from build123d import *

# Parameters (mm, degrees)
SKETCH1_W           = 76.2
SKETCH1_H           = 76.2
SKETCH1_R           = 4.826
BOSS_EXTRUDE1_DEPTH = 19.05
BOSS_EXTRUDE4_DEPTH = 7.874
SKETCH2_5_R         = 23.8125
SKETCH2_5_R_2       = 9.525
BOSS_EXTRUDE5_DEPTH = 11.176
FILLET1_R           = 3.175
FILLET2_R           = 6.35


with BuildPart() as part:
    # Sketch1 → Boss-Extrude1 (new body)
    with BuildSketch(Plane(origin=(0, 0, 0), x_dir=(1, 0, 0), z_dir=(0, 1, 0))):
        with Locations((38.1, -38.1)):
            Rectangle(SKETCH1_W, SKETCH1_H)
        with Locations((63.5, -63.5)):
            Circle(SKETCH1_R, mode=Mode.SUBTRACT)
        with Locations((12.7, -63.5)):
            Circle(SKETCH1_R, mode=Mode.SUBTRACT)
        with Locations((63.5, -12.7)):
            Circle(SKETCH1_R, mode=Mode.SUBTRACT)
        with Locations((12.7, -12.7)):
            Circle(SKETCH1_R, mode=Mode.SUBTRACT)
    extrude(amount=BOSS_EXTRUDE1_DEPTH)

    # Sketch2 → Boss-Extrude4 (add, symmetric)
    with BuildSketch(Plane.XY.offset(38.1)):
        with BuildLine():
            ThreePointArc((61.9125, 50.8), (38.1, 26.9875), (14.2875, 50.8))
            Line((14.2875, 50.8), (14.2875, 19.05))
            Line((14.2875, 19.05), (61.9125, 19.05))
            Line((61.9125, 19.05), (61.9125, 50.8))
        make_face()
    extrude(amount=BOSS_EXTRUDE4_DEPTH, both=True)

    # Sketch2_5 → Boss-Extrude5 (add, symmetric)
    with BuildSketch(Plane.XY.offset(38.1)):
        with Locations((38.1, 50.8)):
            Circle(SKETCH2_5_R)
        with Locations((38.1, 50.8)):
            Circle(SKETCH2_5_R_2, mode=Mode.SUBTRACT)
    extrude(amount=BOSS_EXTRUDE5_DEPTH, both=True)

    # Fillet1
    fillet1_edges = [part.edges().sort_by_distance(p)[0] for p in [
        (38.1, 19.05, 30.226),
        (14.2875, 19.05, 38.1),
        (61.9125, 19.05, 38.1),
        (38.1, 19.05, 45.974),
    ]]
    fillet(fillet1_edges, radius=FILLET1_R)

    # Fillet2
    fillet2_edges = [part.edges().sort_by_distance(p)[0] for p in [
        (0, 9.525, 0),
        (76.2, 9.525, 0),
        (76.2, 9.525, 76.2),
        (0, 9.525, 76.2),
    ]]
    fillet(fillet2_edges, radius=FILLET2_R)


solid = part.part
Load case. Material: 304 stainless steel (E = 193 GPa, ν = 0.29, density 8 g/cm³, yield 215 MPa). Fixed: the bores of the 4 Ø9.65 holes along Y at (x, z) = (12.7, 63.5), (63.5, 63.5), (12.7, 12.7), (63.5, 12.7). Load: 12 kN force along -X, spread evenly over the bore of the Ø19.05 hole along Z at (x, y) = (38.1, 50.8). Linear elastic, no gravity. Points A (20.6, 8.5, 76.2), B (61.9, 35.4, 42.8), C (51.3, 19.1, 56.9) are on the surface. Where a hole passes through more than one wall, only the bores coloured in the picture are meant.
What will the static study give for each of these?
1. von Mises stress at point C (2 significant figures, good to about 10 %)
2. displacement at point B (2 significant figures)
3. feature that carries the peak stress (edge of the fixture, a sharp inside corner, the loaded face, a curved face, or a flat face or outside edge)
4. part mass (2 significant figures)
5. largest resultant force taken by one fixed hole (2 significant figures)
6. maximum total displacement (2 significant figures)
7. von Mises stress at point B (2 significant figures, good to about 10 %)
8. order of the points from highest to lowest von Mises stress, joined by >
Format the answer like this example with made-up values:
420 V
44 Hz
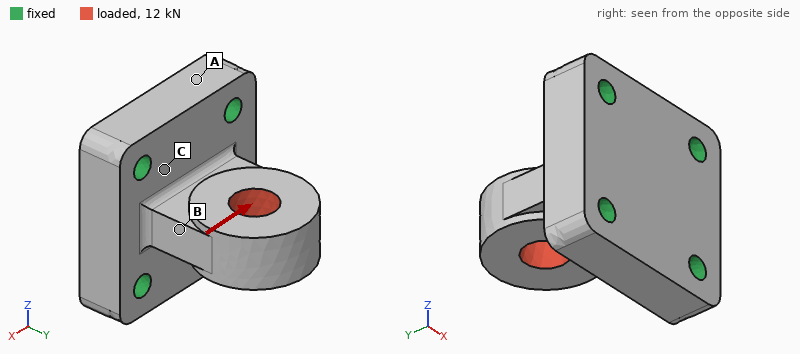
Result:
19 MPa
14 µm
a curved face
1.2 kg
5.8 kN
33 µm
39 MPa
B > C > A
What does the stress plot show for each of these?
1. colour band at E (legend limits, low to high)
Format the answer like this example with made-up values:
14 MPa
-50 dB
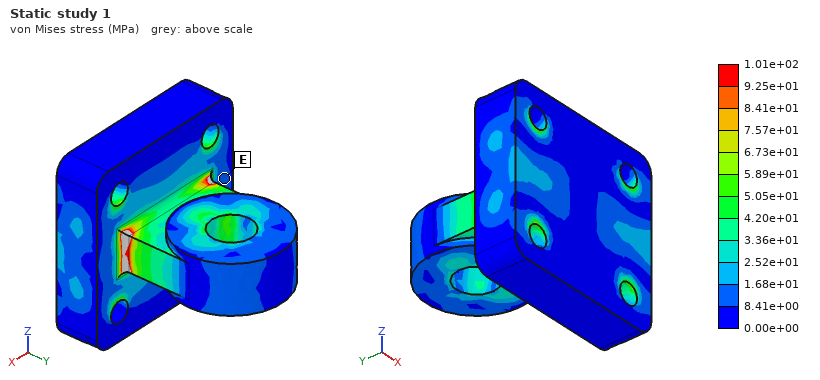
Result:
8.41e+00 to 1.68e+01 MPa
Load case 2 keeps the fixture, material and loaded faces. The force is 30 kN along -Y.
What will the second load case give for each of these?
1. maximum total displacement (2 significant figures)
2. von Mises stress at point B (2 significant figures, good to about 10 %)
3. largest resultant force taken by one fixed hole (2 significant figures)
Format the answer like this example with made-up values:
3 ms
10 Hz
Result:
17 µm
37 MPa
7.7 kN
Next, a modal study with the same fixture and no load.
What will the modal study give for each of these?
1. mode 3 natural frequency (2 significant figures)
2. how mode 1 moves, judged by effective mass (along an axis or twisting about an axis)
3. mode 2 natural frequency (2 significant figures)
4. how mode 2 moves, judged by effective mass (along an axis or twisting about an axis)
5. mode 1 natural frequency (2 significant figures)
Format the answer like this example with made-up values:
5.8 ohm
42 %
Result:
9500 Hz
along Z
6500 Hz
along X
3600 Hz
